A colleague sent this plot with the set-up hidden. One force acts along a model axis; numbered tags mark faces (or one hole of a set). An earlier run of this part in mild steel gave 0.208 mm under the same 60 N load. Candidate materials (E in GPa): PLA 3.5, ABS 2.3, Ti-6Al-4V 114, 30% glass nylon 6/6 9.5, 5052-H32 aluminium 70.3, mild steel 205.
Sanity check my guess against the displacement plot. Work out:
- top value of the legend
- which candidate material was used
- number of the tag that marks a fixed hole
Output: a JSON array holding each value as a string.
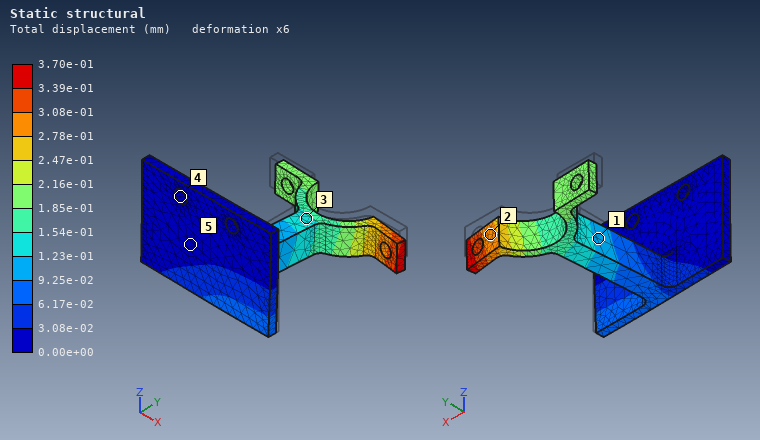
["3.70e-01 mm", "Ti-6Al-4V", "4"]
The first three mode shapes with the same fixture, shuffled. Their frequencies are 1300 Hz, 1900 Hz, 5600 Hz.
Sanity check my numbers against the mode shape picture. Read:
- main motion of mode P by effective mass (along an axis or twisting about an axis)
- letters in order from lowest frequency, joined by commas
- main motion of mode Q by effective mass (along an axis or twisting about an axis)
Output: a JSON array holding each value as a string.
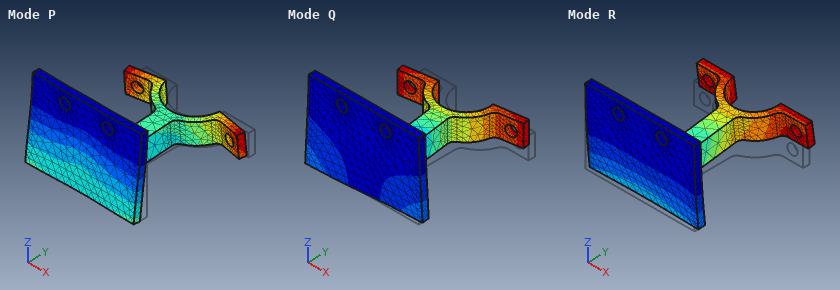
["along Y", "R, Q, P", "along X"]
